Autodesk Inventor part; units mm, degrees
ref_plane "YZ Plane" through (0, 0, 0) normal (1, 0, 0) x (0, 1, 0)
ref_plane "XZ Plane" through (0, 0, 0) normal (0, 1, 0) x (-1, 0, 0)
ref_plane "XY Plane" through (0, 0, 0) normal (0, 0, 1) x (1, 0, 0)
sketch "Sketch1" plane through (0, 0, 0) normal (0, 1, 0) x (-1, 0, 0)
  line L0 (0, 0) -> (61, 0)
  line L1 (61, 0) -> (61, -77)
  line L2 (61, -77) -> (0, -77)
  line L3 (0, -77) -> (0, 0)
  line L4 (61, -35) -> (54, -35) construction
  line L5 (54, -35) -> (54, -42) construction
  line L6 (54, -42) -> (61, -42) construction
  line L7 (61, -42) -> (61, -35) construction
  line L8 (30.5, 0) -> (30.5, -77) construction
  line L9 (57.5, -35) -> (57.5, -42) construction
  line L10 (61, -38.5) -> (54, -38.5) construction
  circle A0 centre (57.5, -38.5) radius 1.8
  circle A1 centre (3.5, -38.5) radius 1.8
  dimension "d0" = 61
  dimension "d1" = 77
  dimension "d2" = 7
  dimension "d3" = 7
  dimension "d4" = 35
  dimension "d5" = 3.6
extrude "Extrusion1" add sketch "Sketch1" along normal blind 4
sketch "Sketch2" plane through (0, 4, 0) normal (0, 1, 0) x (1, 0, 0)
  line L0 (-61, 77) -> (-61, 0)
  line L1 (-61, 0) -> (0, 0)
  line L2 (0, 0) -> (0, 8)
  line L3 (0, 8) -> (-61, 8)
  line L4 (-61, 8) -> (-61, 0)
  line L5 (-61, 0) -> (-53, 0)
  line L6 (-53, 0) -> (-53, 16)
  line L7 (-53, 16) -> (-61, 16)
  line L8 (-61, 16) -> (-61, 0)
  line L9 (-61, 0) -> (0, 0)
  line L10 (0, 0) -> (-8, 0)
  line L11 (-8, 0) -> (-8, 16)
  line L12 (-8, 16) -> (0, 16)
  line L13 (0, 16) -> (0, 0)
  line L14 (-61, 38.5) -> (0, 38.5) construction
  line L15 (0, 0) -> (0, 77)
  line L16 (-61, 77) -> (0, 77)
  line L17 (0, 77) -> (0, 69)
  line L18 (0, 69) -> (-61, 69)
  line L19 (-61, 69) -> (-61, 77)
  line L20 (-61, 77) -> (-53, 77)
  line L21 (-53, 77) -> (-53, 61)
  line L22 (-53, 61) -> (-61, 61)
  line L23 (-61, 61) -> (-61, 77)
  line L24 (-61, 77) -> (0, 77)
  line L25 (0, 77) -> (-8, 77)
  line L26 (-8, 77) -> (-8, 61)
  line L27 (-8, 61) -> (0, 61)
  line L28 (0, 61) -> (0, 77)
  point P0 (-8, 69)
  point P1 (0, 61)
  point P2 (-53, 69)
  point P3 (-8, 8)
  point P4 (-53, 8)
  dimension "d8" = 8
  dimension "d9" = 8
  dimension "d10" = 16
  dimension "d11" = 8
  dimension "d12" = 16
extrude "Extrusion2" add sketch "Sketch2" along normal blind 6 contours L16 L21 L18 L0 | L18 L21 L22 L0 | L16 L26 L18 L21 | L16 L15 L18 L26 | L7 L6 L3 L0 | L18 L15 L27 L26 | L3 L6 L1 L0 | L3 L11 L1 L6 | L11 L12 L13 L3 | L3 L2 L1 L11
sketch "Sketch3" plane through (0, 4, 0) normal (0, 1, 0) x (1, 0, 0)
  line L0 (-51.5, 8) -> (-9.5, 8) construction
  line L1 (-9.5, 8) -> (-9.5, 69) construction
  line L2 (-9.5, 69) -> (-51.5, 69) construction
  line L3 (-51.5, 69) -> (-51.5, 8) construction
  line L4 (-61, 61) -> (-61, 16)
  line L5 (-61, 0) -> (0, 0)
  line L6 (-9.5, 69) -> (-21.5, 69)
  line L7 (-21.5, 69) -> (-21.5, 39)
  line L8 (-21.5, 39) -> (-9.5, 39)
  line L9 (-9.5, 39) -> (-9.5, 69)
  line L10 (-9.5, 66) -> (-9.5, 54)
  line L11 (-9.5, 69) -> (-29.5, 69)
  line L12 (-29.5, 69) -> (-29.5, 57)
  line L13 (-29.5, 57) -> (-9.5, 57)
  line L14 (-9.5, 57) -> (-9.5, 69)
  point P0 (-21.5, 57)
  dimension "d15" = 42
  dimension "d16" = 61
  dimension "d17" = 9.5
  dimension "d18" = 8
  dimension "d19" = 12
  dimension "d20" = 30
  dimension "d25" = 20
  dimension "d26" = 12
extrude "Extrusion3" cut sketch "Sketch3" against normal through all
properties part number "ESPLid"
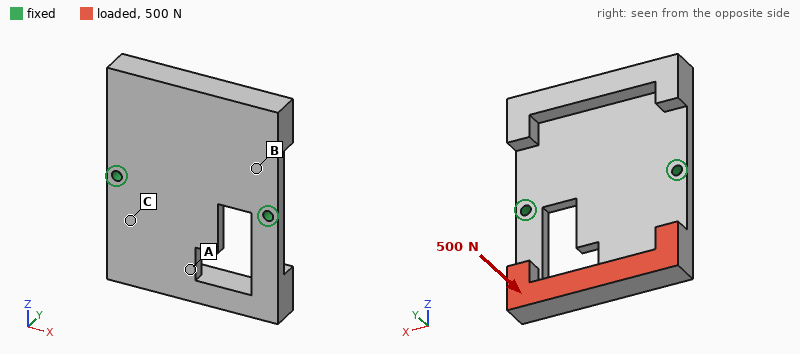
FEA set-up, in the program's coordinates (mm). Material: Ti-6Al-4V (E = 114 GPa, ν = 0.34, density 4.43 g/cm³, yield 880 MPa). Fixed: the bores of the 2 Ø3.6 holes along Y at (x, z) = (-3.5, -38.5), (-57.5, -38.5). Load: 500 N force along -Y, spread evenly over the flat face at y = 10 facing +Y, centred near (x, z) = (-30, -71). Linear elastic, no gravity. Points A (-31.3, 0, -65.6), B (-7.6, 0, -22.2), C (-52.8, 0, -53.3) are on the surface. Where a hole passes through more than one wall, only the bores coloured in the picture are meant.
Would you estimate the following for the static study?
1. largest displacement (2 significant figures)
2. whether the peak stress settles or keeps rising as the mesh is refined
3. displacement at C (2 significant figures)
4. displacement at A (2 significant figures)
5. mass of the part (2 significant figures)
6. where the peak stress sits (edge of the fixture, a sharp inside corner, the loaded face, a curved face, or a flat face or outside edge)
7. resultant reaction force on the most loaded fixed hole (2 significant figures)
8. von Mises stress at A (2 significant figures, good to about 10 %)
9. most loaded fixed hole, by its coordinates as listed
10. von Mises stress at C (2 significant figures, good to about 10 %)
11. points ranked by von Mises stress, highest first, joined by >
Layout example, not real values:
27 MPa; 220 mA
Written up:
0.38 mm; keeps rising; 0.084 mm; 0.22 mm; 110 g; edge of the fixture; 290 N; 43 MPa; (-57.5, -38.5); 74 MPa; C > A > B
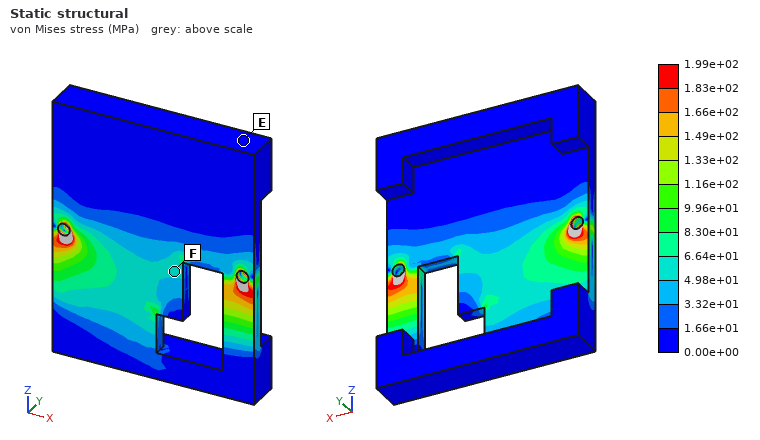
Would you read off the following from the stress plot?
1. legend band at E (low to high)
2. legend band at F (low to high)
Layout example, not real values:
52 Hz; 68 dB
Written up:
0.00e+00 to 1.66e+01 MPa; 4.98e+01 to 6.64e+01 MPa
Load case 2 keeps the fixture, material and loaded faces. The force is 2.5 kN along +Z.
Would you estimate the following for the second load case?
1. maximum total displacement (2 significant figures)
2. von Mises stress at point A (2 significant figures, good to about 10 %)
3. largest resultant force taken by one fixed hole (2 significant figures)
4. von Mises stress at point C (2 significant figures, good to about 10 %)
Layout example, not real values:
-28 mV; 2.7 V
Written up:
0.66 mm; 140 MPa; 1.3 kN; 150 MPa
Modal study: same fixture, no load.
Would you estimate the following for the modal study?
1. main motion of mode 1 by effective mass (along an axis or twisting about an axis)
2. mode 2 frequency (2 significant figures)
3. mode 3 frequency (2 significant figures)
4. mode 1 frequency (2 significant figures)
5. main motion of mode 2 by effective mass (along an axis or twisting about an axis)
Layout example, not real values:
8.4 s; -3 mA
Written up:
twisting about X; 1400 Hz; 3100 Hz; 1100 Hz; along Y
